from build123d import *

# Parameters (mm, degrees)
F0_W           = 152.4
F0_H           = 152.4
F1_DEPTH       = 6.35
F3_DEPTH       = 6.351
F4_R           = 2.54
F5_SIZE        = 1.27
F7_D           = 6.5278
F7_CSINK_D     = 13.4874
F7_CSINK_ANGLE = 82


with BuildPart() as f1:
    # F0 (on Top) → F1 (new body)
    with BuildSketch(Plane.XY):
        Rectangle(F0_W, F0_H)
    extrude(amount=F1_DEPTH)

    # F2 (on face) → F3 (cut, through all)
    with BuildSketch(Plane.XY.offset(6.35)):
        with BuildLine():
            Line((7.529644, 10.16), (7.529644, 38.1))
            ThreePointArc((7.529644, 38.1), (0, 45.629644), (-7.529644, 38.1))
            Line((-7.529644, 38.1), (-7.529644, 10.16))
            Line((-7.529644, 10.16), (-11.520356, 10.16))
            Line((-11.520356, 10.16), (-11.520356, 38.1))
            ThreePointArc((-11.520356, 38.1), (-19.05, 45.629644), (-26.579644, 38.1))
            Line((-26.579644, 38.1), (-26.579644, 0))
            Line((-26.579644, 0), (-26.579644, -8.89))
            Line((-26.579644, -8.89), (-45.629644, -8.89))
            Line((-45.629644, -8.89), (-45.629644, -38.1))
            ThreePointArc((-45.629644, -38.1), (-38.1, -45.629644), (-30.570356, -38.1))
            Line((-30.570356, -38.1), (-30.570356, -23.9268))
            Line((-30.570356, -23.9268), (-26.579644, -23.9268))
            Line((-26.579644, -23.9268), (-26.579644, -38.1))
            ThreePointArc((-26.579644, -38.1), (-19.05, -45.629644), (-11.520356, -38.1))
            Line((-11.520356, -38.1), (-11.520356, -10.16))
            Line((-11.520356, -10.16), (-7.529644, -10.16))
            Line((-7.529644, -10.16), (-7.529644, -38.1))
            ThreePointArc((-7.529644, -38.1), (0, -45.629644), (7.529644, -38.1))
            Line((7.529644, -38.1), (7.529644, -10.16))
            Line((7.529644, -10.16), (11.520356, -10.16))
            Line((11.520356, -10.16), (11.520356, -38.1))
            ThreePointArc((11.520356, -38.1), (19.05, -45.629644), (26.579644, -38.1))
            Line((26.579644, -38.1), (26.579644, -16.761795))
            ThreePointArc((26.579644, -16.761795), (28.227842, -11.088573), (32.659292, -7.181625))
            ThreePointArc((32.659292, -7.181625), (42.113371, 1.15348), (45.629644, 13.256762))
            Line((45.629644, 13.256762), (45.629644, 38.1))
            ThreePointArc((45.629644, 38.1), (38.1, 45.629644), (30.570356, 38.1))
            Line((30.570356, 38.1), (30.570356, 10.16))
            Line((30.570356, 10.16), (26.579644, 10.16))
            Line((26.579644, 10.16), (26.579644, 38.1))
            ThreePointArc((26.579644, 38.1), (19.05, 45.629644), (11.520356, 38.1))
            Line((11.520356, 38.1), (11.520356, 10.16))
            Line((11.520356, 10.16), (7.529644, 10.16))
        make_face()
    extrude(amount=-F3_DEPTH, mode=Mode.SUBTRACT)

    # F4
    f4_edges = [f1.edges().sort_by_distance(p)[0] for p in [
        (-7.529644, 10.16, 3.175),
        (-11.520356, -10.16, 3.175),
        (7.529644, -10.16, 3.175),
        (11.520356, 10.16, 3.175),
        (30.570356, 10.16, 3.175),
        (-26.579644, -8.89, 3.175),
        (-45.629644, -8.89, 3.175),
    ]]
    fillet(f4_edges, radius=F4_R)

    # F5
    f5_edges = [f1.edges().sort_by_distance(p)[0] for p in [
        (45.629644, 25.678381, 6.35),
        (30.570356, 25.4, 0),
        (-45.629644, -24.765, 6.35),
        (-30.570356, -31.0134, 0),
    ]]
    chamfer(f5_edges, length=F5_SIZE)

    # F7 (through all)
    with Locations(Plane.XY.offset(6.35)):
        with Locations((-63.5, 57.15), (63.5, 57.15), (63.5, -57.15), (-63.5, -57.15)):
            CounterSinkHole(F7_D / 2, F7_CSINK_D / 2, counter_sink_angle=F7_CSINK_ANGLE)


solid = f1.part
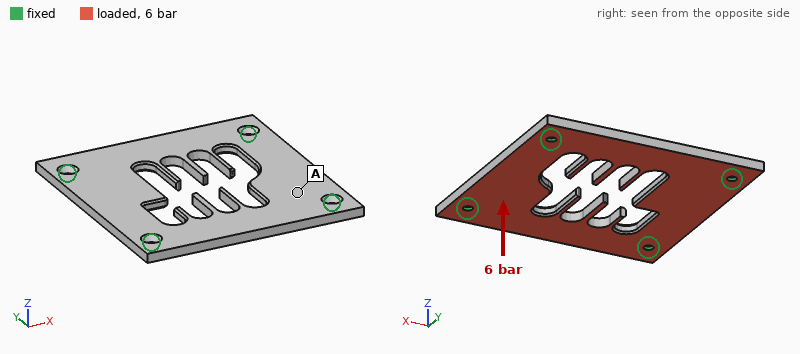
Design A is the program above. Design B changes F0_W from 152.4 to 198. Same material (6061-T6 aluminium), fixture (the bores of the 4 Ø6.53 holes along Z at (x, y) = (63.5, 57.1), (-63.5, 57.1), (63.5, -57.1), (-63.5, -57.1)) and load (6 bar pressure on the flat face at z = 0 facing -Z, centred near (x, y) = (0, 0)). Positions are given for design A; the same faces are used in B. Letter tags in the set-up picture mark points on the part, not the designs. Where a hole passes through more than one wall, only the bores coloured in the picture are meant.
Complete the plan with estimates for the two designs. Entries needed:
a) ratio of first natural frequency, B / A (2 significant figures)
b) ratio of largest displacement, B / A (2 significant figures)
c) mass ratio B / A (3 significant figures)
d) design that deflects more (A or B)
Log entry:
0.96
0.84
1.40
A
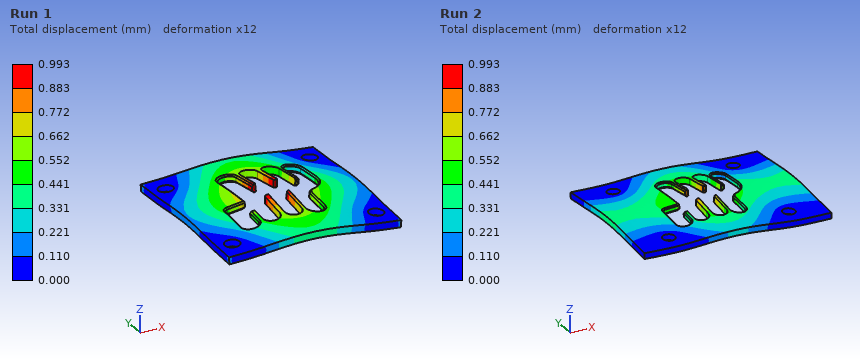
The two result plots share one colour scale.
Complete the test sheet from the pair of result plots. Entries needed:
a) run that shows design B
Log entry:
Run 2
